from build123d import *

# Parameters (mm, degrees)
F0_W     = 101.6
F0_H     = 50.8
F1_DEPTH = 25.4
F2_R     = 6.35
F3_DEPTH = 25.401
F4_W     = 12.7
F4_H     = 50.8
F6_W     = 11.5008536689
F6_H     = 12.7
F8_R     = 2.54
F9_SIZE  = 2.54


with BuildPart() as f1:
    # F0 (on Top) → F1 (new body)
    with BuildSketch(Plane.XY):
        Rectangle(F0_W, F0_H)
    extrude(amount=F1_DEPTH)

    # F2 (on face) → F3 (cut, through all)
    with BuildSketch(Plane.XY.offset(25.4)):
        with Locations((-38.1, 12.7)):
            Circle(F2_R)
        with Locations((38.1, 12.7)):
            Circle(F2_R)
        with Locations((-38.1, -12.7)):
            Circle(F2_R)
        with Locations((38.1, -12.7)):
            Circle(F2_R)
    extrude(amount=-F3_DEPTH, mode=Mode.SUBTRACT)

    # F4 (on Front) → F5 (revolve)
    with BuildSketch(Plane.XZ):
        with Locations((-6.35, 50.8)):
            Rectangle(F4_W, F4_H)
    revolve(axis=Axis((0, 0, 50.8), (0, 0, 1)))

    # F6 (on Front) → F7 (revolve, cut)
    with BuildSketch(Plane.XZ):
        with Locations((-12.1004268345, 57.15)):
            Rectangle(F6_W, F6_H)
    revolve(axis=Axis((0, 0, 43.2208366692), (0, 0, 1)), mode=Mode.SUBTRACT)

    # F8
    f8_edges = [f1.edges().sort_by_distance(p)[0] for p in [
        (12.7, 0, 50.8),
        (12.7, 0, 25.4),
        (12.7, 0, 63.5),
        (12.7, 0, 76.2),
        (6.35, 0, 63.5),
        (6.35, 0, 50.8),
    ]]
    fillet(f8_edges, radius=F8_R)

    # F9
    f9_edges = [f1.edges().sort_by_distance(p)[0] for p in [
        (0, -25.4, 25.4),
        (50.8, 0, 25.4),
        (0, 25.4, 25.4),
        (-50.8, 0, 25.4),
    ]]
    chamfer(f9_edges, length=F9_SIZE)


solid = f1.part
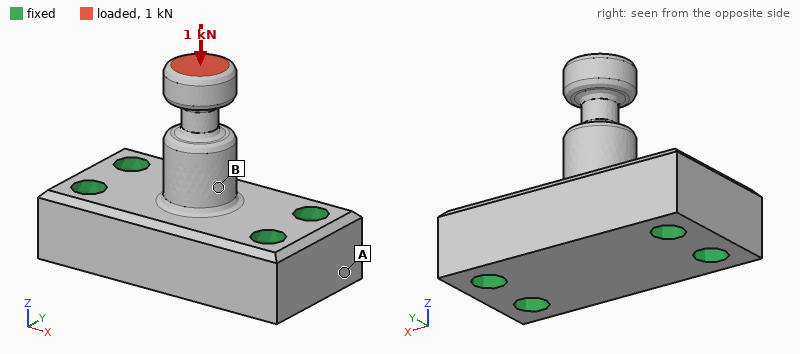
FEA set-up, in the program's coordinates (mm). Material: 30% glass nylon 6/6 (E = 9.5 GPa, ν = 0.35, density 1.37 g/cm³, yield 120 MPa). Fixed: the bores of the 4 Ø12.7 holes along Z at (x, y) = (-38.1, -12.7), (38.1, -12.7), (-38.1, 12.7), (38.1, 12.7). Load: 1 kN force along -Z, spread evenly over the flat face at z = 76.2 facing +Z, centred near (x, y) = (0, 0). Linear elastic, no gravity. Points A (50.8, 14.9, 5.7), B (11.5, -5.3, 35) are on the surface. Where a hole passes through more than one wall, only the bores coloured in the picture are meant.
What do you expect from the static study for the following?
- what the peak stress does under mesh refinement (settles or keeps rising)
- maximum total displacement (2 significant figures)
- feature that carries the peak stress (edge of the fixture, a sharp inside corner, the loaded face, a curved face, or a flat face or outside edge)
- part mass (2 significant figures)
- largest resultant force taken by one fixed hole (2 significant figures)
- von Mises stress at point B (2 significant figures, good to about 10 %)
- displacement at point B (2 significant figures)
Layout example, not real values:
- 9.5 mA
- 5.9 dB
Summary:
- keeps rising
- 28 µm
- a sharp inside corner
- 190 g
- 260 N
- 1.9 MPa
- 7.8 µm
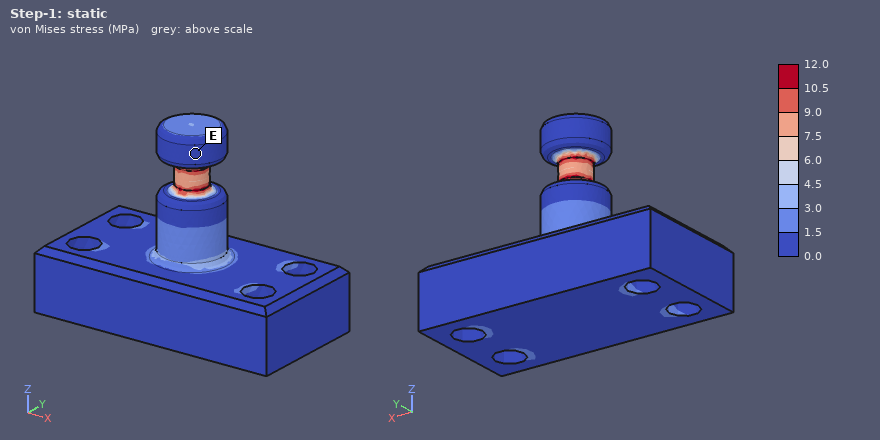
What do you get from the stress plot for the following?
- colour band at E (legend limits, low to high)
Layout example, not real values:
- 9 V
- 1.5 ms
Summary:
- 0.0 to 1.5 MPa
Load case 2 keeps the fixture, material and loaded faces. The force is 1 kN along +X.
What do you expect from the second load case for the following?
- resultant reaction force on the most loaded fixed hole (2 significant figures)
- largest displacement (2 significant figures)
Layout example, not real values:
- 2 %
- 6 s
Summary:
- 620 N
- 0.83 mm
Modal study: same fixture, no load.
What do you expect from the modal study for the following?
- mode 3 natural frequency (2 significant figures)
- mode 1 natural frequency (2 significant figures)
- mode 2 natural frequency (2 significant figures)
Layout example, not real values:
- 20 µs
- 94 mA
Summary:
- 4600 Hz
- 2200 Hz
- 2300 Hz
